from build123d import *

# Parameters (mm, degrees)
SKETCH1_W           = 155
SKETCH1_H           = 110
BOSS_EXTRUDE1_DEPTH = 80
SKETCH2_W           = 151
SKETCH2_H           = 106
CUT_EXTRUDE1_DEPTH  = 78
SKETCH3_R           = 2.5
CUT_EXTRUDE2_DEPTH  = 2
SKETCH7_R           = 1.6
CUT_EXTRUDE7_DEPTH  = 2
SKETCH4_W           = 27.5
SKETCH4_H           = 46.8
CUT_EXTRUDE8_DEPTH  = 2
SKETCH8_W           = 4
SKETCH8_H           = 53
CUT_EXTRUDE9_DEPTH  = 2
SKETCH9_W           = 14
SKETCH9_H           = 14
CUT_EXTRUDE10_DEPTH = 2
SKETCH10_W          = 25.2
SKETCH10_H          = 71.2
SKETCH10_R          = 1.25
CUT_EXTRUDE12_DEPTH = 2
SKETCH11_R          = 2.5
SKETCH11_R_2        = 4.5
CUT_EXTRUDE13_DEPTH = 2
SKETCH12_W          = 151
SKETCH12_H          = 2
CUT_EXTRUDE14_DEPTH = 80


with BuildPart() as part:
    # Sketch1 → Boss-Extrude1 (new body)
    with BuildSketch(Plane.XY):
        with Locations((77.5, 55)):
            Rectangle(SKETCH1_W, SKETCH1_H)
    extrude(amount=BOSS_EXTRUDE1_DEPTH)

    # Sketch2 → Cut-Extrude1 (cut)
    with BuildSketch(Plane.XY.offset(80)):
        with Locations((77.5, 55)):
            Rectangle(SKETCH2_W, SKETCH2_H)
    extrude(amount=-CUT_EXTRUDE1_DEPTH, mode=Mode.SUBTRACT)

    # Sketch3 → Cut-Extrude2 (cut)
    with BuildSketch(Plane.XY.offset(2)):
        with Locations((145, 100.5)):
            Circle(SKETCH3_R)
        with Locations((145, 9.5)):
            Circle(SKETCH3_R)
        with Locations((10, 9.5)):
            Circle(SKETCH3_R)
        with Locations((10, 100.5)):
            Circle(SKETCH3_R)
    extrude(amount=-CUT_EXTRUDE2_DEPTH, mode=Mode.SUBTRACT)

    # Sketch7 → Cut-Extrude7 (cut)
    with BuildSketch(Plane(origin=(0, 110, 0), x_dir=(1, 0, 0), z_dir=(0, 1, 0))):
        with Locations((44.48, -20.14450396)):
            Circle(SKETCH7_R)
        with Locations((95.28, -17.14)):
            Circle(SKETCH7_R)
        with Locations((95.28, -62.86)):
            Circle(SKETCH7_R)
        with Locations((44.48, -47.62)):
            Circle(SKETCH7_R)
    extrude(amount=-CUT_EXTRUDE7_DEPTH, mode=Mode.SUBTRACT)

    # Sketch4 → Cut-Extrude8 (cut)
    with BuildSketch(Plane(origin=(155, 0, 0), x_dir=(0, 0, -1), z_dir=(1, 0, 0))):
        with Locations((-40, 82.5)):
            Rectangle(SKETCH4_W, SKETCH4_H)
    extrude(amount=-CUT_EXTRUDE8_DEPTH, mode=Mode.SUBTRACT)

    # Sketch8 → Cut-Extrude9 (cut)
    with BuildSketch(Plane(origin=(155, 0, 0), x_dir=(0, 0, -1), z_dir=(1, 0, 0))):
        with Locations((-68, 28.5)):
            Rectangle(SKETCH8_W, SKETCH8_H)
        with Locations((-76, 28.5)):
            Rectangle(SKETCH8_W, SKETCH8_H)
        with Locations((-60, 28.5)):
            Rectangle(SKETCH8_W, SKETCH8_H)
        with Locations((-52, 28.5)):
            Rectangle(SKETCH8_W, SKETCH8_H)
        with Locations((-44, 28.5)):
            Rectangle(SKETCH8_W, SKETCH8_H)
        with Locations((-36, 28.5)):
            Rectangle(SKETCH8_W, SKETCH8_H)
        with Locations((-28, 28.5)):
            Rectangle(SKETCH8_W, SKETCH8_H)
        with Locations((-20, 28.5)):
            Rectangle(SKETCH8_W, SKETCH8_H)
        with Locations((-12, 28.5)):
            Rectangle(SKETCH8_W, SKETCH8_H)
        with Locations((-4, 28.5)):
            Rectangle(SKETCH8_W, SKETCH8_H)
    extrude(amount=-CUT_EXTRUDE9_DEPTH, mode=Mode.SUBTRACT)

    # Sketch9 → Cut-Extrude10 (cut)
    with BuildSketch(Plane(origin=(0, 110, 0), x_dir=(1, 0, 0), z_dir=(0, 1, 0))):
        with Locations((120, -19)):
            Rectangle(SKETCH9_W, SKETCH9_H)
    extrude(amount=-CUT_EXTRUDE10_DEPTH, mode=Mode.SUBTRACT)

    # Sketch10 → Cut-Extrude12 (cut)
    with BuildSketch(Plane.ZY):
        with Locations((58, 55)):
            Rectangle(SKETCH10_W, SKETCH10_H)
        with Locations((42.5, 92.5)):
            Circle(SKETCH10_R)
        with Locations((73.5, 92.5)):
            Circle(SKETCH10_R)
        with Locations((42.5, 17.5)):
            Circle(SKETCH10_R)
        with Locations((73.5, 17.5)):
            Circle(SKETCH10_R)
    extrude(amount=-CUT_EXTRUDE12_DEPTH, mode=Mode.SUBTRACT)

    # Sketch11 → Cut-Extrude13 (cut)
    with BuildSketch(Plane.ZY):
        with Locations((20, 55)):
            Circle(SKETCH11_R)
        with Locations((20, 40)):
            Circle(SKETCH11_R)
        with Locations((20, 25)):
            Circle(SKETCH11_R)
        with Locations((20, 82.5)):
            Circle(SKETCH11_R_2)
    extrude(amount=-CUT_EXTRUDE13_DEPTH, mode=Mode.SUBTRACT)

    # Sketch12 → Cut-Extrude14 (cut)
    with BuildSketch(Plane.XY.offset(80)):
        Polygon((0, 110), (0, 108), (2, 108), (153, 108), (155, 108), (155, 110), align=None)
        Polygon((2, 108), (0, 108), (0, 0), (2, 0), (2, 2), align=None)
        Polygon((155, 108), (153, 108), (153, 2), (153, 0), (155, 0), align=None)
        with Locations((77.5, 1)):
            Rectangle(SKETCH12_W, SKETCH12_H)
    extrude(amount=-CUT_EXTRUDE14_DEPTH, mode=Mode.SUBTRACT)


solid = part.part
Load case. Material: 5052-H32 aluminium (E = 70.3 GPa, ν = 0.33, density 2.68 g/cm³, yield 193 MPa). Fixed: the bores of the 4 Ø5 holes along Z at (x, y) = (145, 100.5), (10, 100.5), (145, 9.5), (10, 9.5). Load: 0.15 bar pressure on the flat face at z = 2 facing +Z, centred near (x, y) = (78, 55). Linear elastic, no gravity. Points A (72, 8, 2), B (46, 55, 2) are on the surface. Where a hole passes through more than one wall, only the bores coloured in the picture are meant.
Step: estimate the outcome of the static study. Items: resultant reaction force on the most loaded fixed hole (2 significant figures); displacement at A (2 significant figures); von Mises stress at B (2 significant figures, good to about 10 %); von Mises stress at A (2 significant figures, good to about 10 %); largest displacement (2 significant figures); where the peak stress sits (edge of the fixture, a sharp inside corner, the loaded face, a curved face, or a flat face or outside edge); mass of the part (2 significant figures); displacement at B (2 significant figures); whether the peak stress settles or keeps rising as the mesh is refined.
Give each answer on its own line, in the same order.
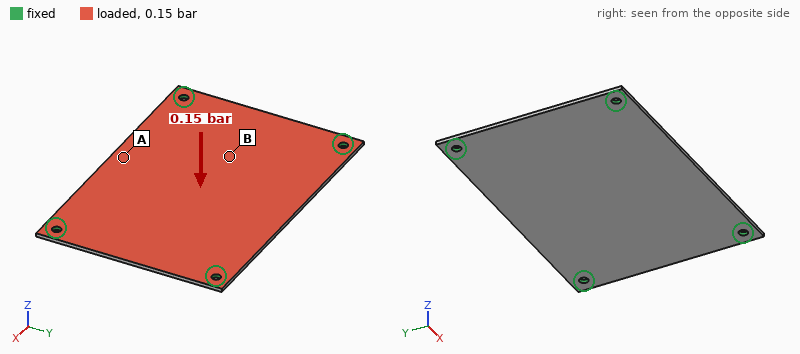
60 N
0.37 mm
12 MPa
22 MPa
0.42 mm
edge of the fixture
85 g
0.32 mm
keeps rising
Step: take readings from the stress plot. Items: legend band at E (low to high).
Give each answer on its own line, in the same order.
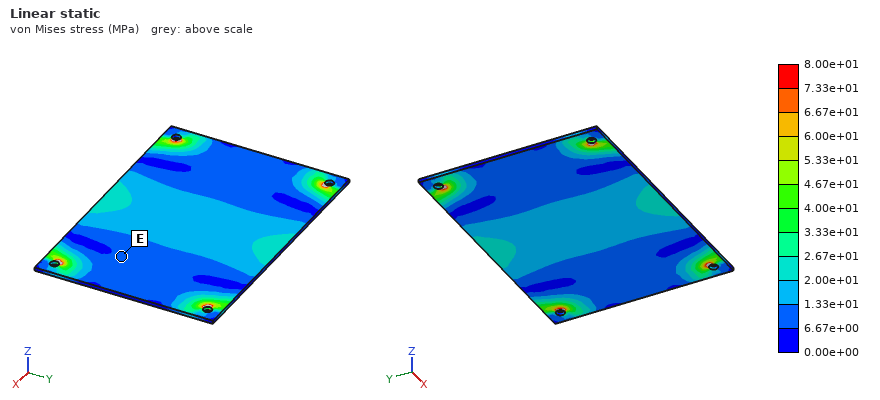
6.67e+00 to 1.33e+01 MPa
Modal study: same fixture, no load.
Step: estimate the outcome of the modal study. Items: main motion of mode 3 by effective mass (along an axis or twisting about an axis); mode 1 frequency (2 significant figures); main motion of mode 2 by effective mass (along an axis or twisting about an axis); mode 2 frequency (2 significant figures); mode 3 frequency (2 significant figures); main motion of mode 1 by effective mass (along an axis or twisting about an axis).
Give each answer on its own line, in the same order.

twisting about Y
480 Hz
twisting about X
760 Hz
1200 Hz
along Z
